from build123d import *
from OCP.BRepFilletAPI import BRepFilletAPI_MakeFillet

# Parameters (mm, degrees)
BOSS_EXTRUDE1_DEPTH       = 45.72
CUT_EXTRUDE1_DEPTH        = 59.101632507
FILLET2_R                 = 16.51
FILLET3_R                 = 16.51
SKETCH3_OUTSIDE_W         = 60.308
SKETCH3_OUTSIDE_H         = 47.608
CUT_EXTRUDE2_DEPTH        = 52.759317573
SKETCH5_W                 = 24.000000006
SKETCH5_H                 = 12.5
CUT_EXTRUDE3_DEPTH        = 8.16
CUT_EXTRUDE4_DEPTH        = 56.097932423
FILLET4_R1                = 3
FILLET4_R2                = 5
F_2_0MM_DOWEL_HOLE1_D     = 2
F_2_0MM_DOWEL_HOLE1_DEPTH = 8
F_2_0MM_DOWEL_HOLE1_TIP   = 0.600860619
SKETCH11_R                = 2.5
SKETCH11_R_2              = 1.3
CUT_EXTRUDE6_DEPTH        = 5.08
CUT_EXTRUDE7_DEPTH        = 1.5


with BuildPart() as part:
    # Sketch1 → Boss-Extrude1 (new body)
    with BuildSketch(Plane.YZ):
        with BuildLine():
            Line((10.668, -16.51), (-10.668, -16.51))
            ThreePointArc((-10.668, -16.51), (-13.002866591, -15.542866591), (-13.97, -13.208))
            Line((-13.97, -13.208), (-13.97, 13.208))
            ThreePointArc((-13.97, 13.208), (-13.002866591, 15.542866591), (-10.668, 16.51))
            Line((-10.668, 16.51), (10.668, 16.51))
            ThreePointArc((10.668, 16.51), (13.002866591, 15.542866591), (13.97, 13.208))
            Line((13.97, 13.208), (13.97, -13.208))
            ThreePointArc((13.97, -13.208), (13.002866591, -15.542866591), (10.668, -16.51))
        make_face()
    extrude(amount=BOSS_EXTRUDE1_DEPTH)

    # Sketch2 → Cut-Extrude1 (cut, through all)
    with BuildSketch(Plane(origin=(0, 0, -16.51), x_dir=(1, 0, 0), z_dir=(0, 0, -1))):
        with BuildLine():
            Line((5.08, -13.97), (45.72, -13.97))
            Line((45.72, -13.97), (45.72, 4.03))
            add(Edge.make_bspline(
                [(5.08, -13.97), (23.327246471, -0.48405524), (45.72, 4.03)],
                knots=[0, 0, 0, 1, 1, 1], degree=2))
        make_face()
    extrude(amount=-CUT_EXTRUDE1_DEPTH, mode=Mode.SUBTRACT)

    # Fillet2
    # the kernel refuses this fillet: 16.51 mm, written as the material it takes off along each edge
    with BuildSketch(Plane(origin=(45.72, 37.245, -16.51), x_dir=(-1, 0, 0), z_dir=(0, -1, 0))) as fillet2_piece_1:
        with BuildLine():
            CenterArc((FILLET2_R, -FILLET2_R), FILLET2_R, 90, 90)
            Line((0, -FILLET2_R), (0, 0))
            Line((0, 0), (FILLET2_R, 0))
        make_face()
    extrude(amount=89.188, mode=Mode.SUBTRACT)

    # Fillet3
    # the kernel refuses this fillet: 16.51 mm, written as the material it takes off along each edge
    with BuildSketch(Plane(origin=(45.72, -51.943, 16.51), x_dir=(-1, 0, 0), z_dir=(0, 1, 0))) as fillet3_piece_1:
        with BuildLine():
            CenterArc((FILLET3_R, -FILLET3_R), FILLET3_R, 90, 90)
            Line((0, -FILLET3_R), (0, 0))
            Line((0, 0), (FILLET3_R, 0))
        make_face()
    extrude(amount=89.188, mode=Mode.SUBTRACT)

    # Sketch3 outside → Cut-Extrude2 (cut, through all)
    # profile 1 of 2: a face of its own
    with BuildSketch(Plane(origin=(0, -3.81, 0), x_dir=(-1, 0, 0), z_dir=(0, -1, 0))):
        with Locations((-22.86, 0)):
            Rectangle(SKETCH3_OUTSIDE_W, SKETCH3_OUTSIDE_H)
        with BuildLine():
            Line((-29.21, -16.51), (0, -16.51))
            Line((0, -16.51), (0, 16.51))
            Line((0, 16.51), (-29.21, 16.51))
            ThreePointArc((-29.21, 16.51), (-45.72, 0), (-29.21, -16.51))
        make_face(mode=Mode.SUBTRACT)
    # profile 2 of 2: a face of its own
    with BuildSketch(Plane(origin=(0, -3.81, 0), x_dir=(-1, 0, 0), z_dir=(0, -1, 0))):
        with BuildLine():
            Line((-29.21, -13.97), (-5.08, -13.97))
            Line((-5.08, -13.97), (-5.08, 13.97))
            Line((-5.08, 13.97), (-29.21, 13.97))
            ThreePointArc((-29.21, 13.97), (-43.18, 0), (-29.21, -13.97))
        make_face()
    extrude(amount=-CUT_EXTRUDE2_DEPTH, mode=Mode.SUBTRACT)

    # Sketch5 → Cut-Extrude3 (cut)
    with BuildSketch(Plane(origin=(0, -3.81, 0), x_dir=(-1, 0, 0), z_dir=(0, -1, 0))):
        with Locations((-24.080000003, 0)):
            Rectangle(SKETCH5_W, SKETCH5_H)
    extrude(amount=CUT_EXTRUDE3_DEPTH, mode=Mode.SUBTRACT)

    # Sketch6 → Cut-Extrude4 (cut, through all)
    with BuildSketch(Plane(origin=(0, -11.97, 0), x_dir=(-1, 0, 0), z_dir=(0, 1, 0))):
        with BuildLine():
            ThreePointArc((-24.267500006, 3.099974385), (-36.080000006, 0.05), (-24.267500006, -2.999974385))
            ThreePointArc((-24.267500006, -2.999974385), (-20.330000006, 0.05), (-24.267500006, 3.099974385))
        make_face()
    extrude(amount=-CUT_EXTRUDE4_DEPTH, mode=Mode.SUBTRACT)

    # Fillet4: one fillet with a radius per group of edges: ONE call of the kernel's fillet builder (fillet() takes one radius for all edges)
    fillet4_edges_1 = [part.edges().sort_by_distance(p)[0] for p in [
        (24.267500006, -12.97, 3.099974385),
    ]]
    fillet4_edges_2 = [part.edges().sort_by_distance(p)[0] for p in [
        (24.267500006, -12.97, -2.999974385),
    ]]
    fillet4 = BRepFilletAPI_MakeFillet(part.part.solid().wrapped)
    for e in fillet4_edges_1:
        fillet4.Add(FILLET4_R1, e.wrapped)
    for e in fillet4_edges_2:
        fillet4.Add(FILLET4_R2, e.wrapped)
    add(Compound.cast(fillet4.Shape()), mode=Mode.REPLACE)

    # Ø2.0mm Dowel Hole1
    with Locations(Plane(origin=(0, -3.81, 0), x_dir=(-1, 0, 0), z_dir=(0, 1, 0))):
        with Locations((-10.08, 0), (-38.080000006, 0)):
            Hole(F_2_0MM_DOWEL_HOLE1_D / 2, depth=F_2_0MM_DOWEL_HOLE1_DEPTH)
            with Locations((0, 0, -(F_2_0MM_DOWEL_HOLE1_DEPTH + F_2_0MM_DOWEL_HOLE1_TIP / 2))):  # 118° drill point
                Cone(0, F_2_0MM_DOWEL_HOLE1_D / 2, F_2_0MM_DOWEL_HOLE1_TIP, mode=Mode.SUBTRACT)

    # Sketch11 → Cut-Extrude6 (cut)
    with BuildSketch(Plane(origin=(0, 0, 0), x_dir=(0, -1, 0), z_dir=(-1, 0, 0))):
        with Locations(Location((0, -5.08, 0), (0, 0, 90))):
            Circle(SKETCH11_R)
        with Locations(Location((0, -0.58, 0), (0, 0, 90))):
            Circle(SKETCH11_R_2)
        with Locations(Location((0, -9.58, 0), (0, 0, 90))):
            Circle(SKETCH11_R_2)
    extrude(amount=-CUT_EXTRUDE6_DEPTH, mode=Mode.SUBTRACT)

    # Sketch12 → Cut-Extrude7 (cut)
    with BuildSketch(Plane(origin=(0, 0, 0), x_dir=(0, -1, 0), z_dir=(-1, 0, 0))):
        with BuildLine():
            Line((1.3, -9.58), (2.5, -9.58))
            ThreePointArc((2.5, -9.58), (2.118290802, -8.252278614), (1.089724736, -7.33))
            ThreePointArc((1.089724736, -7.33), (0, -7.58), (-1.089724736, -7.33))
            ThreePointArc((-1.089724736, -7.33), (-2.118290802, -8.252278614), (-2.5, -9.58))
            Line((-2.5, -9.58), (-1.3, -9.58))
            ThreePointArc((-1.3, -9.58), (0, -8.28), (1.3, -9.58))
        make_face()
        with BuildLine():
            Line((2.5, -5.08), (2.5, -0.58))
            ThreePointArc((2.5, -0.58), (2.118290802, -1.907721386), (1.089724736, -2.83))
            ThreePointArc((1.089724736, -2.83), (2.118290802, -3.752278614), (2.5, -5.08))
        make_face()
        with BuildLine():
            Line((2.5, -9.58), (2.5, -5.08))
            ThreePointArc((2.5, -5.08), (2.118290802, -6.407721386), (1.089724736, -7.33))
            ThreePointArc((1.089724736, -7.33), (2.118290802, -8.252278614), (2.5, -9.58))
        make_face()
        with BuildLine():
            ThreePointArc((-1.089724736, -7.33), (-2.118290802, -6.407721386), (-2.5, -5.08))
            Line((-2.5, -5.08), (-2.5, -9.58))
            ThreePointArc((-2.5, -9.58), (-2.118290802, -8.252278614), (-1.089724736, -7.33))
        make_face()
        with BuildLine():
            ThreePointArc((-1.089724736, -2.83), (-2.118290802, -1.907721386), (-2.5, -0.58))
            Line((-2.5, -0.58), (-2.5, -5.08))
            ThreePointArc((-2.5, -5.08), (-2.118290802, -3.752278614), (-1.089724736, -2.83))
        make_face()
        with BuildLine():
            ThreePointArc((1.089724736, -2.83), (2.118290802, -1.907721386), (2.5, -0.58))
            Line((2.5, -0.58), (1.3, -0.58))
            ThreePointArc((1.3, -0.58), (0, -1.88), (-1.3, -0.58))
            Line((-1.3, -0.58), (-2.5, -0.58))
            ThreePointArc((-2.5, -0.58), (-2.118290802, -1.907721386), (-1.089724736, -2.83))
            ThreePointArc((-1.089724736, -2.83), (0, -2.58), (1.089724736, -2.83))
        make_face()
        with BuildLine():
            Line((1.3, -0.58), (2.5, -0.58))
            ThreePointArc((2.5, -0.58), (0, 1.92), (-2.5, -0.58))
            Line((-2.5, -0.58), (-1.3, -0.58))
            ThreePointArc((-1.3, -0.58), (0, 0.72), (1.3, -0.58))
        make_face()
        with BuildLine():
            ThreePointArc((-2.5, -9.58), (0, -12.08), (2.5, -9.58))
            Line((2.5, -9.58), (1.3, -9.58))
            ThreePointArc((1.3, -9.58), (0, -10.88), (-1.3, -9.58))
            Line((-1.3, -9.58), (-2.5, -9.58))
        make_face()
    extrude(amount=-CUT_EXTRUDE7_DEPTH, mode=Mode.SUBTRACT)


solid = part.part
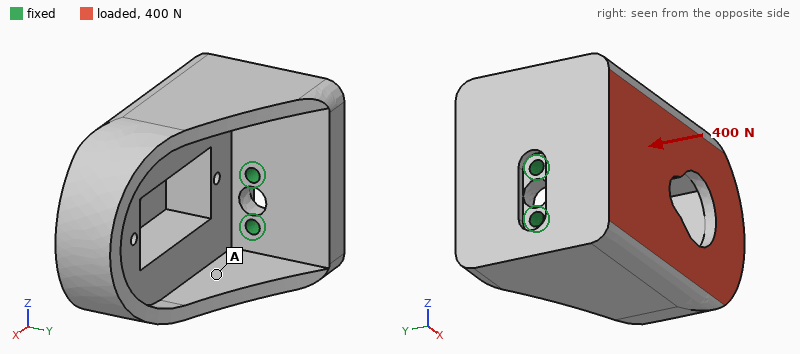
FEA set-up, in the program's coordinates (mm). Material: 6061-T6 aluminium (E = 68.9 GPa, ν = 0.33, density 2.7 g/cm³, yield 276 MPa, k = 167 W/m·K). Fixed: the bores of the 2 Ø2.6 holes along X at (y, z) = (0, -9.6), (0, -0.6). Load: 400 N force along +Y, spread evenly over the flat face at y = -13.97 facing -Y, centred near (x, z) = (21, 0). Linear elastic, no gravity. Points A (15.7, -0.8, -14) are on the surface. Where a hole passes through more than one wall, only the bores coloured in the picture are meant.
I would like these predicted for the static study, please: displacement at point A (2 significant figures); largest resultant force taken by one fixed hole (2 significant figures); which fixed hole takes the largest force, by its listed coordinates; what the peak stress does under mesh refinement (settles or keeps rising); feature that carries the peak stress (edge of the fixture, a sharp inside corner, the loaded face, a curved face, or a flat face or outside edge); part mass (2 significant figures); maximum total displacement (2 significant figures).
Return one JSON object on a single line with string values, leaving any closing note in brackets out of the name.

{"displacement at point A": "0.032 mm", "largest resultant force taken by one fixed hole": "390 N", "which fixed hole takes the largest force, by its listed coordinates": "(0, -0.6)", "what the peak stress does under mesh refinement": "keeps rising", "feature that carries the peak stress": "edge of the fixture", "part mass": "42 g", "maximum total displacement": "0.13 mm"}
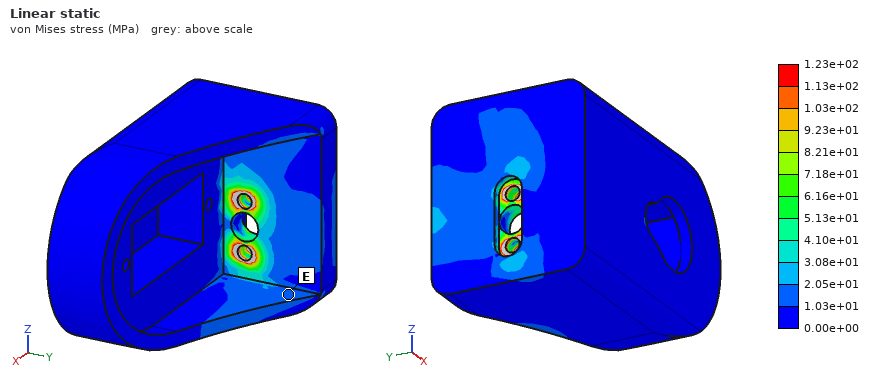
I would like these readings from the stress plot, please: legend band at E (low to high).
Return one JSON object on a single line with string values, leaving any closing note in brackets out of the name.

{"legend band at E": "1.03e+01 to 2.05e+01 MPa"}
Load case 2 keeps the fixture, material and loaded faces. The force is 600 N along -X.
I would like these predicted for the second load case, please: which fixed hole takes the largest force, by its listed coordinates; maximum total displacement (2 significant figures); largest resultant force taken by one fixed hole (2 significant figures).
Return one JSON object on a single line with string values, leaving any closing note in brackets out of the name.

{"which fixed hole takes the largest force, by its listed coordinates": "(0, -0.6)", "maximum total displacement": "0.13 mm", "largest resultant force taken by one fixed hole": "530 N"}
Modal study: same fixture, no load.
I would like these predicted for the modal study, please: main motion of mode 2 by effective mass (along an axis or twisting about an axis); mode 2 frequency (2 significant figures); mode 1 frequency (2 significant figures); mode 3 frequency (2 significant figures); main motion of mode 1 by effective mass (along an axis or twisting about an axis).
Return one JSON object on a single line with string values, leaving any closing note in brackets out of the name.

{"main motion of mode 2 by effective mass": "along Z", "mode 2 frequency": "3000 Hz", "mode 1 frequency": "1900 Hz", "mode 3 frequency": "7200 Hz", "main motion of mode 1 by effective mass": "along Y"}
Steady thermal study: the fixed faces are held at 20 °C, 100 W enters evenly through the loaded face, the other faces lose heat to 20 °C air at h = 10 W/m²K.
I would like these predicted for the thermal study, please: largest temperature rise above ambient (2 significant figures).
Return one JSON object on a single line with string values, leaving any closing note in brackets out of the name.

{"largest temperature rise above ambient": "75 K"}
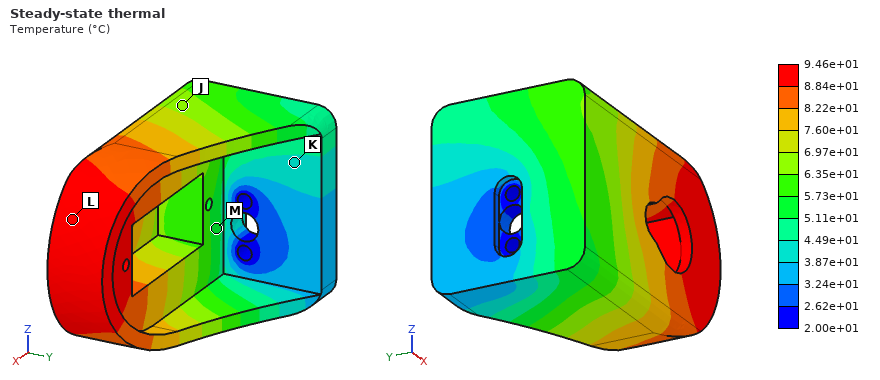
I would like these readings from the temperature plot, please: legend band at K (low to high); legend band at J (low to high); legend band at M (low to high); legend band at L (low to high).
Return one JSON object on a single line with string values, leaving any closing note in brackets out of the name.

{"legend band at K": "3.87e+01 to 4.49e+01 °C", "legend band at J": "6.35e+01 to 6.97e+01 °C", "legend band at M": "5.11e+01 to 5.73e+01 °C", "legend band at L": "8.84e+01 to 9.46e+01 °C"}
